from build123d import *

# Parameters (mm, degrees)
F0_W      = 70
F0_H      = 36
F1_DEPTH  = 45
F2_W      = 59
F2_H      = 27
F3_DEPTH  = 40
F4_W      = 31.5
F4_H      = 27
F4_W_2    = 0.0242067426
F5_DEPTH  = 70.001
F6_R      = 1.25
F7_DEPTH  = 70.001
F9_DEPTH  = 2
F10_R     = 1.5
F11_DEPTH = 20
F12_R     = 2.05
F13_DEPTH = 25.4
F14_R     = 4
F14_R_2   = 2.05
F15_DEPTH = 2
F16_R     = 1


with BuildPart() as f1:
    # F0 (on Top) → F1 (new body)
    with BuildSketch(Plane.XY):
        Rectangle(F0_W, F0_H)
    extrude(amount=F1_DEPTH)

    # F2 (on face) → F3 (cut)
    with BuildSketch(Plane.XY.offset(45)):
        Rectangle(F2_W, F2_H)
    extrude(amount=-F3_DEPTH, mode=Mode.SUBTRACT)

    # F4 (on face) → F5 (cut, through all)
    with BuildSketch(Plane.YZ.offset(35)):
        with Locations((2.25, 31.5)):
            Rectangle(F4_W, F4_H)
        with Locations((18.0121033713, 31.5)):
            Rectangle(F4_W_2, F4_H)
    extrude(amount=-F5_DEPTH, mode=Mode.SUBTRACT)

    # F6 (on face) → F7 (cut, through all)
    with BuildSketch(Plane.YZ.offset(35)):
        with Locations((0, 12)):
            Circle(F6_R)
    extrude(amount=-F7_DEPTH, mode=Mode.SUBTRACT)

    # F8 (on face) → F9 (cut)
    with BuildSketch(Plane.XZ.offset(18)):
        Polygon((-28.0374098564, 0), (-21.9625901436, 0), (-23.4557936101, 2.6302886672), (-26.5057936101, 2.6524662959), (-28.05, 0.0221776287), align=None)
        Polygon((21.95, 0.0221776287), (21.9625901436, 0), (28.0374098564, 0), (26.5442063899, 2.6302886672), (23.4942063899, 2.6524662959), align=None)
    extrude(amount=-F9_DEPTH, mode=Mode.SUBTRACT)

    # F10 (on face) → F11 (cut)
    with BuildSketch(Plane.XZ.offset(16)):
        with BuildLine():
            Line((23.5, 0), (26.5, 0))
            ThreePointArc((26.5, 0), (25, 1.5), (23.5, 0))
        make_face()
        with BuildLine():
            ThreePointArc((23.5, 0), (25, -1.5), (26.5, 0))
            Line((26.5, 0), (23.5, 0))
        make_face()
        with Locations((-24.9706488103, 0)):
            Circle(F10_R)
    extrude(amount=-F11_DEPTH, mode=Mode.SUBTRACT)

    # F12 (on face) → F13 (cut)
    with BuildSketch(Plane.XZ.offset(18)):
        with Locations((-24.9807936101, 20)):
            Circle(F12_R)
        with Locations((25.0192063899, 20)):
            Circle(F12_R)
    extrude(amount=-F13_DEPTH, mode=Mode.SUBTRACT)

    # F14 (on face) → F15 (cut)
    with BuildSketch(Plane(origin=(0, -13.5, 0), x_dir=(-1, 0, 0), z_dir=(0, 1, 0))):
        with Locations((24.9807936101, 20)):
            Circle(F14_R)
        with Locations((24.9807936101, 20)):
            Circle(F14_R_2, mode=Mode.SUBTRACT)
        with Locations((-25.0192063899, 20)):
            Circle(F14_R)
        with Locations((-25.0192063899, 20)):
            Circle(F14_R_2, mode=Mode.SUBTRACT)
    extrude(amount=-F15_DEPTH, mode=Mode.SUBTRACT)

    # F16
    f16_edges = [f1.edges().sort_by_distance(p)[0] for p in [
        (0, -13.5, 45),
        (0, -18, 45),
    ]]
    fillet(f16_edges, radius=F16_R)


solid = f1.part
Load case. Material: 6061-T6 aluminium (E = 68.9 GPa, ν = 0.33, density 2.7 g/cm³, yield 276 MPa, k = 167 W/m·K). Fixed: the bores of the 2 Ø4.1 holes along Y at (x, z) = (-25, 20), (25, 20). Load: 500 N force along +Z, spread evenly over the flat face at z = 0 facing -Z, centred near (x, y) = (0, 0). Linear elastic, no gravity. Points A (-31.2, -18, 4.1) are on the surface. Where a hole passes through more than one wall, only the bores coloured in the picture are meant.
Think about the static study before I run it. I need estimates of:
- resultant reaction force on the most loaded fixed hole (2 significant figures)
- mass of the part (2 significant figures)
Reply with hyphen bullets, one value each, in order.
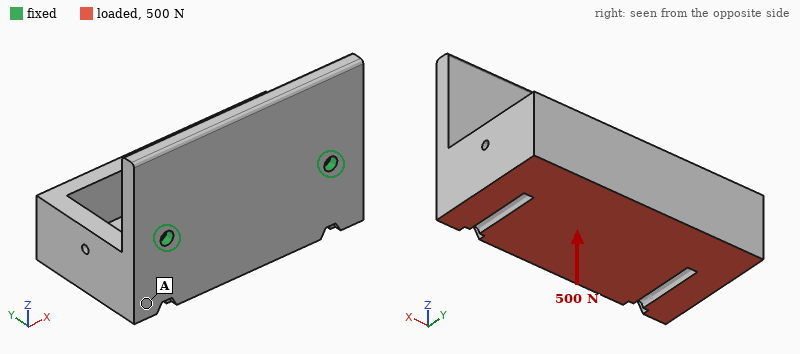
- 260 N
- 88 g
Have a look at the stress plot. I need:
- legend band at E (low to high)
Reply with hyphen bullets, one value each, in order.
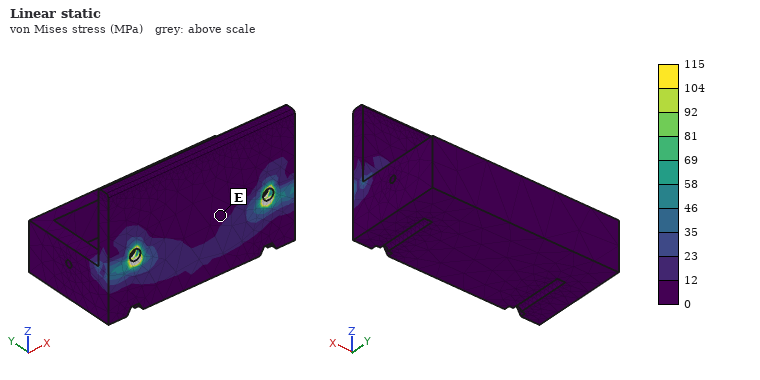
- 0 to 12 MPa
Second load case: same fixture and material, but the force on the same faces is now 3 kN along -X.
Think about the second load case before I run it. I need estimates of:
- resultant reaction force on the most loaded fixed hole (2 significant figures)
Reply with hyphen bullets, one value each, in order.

- 2.1 kN
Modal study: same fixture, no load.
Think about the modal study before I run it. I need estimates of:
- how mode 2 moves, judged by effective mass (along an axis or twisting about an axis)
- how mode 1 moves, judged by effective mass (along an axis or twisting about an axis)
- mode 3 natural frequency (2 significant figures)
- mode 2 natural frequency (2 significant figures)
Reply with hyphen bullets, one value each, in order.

- along X
- along Z
- 3900 Hz
- 2400 Hz
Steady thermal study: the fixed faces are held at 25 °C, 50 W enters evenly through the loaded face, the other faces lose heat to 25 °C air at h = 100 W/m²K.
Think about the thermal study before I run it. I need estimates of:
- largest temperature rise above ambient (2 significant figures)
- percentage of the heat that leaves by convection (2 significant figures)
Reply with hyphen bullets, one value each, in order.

- 22 K
- 34 %
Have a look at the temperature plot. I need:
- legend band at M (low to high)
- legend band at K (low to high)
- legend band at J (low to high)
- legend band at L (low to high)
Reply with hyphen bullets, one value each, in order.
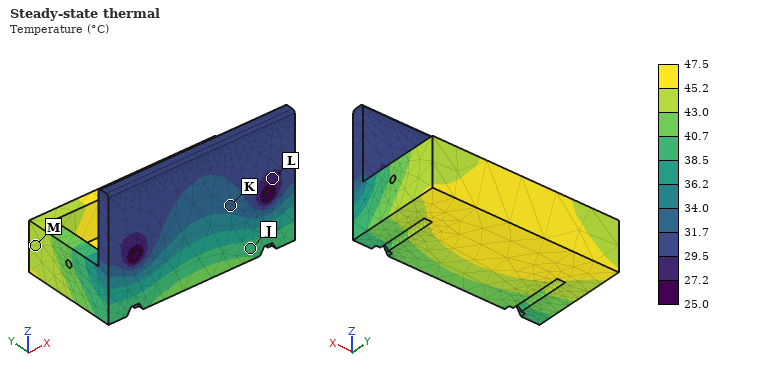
- 43.0 to 45.2 °C
- 31.7 to 34.0 °C
- 38.5 to 40.7 °C
- 27.2 to 29.5 °C
